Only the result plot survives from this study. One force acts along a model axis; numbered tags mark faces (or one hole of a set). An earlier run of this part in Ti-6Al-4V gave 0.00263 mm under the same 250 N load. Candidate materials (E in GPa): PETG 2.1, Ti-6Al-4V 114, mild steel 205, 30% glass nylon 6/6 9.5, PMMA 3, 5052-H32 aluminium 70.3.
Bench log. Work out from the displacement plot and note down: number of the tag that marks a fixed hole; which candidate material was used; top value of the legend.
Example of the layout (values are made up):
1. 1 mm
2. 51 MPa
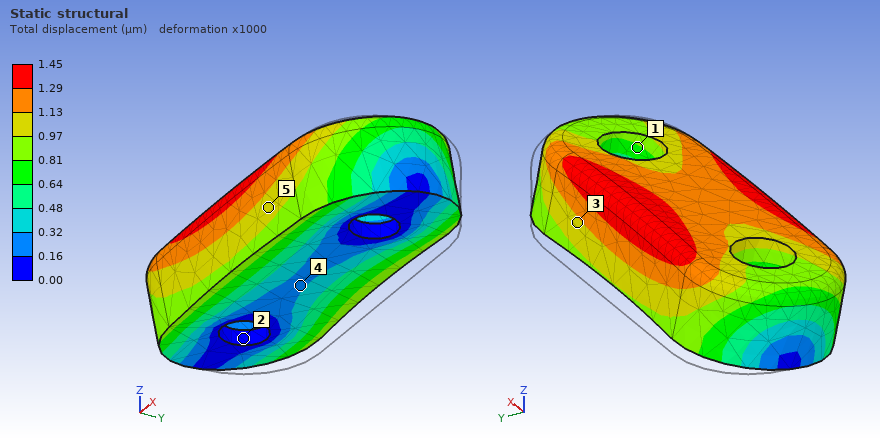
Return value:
1. 2
2. mild steel
3. 1.45 µm
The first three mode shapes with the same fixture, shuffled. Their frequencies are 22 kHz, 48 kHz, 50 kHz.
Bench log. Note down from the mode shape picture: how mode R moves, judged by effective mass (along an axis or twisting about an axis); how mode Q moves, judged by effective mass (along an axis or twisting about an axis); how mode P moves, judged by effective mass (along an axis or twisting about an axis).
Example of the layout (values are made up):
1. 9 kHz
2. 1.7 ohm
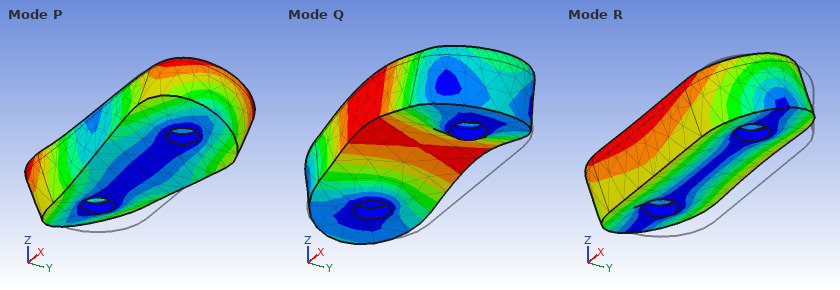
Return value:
1. along Y
2. along Z
3. twisting about Z
